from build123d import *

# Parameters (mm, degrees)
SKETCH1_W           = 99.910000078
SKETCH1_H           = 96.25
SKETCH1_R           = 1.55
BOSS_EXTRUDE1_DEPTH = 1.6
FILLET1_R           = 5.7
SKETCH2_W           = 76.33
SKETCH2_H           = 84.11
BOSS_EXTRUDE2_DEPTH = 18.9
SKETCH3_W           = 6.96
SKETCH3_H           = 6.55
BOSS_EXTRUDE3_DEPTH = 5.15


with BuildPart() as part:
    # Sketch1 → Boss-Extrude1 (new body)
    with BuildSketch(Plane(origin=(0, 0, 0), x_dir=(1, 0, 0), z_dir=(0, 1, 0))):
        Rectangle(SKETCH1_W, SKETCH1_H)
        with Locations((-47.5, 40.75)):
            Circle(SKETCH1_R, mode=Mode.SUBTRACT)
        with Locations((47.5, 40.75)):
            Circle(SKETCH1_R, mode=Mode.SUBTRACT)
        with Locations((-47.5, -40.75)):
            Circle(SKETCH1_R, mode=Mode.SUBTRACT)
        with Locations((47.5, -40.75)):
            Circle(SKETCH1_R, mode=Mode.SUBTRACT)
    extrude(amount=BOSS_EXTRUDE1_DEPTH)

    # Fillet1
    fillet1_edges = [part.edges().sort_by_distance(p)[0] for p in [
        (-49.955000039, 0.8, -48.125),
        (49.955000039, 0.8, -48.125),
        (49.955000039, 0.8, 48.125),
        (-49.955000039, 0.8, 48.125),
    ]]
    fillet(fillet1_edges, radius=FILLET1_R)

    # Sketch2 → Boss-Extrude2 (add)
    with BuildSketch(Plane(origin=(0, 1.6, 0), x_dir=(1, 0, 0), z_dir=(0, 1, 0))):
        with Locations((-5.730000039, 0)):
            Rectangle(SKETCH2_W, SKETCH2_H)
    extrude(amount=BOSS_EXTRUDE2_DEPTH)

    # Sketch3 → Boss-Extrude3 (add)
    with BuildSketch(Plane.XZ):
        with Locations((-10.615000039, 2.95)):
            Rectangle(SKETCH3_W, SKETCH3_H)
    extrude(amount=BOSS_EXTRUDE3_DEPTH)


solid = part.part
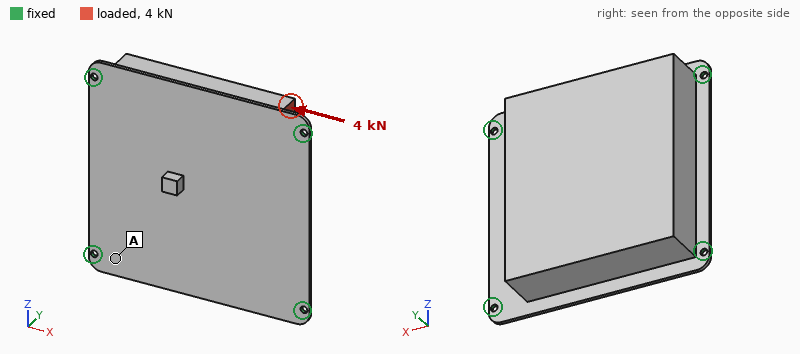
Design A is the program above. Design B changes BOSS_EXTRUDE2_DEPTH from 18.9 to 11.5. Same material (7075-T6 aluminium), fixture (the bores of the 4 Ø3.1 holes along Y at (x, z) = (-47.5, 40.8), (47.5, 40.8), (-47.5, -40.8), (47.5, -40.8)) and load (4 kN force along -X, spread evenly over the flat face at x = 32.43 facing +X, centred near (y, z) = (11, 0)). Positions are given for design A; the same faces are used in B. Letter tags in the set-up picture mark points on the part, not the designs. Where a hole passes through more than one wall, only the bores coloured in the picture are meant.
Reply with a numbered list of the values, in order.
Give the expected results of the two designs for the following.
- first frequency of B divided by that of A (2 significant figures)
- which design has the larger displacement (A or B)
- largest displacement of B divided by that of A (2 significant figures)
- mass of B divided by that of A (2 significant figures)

1. 1.2
2. A
3. 0.63
4. 0.65
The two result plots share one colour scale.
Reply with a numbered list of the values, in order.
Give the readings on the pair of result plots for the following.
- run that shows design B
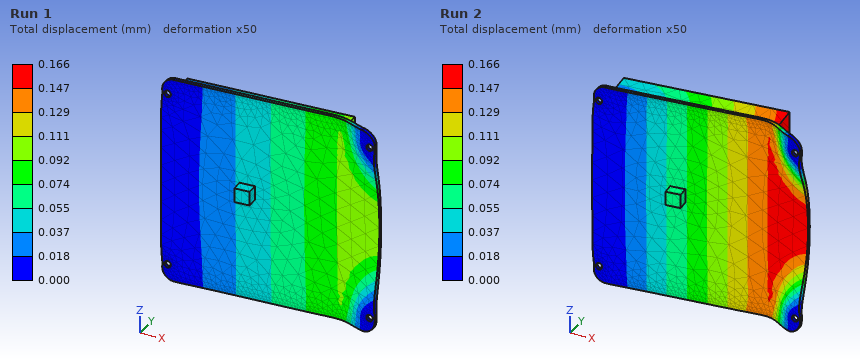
1. Run 1
